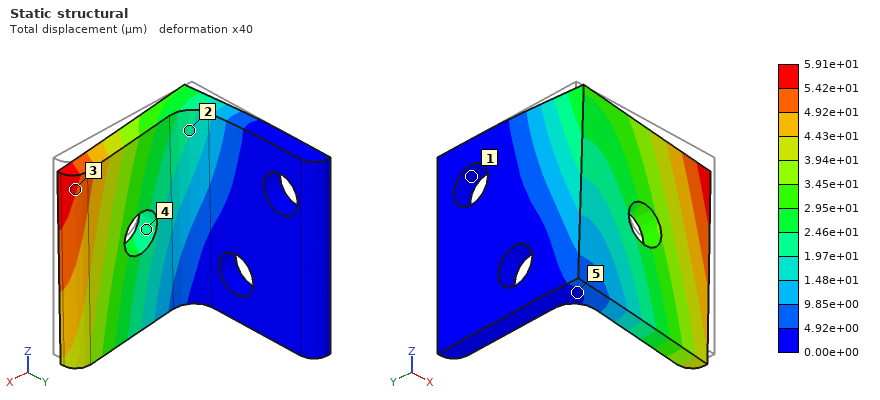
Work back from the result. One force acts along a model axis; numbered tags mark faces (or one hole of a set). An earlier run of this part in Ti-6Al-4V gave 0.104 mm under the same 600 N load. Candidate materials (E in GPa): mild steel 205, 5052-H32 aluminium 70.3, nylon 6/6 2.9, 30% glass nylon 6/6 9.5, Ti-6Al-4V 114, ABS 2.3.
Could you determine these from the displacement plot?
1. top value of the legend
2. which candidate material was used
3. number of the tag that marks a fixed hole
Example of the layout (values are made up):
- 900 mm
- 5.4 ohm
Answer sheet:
- 5.91e+01 µm
- mild steel
- 1
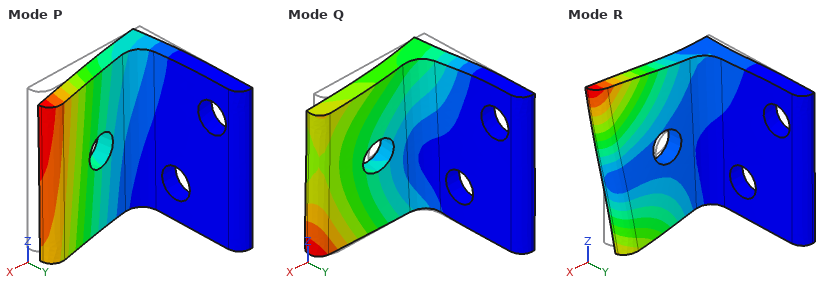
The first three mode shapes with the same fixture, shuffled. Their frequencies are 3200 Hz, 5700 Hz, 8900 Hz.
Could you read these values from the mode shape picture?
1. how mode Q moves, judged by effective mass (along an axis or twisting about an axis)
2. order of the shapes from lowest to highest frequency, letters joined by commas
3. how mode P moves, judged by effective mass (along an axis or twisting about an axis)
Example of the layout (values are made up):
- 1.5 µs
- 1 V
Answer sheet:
- along Z
- P, Q, R
- along Y
